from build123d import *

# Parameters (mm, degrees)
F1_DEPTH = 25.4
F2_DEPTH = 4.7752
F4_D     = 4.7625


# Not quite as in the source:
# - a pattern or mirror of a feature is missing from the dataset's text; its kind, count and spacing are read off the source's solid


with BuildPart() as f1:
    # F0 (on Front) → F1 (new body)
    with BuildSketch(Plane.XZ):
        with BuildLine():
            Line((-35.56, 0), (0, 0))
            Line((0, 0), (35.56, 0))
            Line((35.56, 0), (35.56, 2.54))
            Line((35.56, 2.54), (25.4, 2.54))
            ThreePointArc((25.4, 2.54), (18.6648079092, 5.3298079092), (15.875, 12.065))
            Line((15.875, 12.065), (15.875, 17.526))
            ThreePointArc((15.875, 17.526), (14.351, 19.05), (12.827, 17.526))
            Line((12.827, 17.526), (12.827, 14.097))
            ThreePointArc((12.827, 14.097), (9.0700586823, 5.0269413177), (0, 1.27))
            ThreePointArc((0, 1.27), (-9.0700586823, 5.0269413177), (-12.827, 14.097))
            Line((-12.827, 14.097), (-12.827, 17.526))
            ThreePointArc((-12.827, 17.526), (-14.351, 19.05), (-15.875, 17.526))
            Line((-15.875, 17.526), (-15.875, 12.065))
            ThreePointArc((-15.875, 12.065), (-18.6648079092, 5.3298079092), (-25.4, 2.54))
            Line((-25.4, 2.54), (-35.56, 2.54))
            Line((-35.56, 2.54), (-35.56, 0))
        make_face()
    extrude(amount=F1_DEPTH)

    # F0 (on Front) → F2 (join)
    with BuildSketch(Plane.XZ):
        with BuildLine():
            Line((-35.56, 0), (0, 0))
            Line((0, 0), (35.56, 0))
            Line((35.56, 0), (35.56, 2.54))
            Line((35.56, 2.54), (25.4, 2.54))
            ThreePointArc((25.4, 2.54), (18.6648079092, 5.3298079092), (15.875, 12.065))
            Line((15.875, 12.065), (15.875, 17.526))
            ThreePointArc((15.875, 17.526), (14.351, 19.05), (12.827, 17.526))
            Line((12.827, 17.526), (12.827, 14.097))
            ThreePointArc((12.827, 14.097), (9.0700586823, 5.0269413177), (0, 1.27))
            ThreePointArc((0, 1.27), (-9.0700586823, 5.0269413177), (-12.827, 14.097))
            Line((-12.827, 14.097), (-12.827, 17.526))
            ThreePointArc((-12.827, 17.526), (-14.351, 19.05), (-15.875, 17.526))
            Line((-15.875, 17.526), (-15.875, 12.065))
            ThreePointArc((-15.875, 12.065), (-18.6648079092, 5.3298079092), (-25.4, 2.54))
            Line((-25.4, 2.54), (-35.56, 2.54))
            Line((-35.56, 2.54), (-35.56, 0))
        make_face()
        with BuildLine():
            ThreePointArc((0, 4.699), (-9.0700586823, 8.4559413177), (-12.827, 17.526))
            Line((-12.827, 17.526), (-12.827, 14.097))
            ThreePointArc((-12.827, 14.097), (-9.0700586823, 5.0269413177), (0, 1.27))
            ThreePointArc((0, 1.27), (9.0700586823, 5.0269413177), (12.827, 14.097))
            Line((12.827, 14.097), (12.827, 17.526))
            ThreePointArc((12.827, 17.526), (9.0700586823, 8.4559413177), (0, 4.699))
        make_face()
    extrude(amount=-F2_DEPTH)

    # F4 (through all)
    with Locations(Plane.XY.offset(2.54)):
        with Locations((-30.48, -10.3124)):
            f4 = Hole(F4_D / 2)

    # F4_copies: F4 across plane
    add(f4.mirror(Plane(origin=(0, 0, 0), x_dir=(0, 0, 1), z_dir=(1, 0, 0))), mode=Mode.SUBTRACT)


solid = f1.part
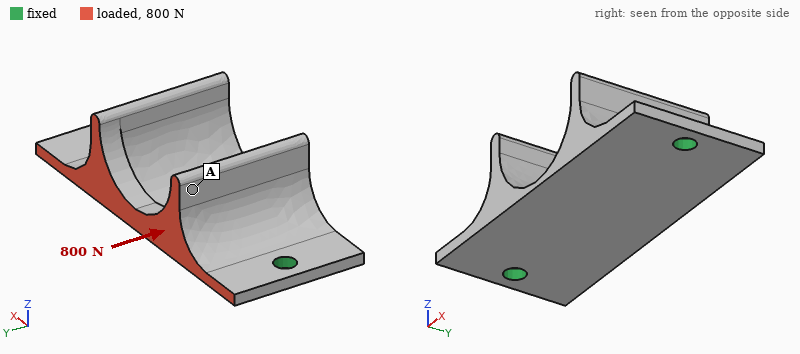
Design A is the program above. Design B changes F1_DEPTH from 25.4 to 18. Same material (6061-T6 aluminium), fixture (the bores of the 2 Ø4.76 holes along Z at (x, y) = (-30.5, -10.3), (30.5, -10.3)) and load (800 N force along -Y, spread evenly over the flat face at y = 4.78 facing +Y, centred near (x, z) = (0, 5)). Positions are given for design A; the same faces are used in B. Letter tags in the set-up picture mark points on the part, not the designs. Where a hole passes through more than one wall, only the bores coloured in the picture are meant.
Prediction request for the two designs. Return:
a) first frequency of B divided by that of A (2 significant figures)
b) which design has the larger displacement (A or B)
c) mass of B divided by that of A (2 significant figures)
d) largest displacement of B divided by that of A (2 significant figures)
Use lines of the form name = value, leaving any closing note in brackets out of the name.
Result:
first frequency of B divided by that of A = 0.99
which design has the larger displacement = B
mass of B divided by that of A = 0.76
largest displacement of B divided by that of A = 1.3
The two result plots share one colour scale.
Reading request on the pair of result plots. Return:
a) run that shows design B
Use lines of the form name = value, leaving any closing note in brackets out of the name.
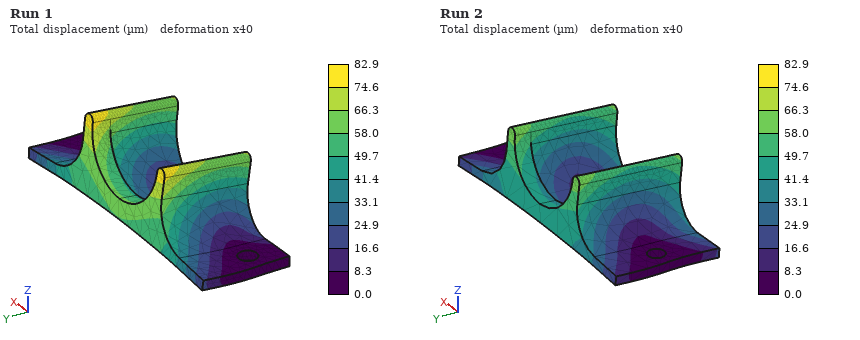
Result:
run that shows design B = Run 1
